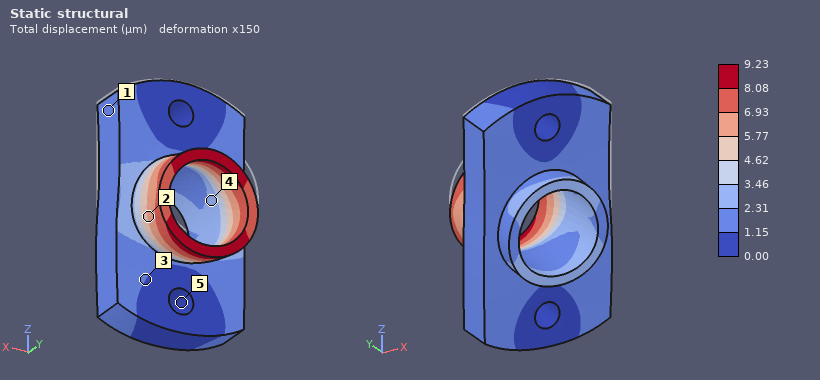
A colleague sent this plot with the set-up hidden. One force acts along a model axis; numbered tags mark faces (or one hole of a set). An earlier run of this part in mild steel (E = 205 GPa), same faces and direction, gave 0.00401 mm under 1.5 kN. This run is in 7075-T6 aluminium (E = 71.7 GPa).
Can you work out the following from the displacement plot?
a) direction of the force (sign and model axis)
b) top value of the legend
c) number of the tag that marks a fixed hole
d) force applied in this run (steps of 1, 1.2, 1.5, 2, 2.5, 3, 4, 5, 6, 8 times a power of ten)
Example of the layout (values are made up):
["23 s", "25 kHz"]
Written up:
["-Z", "9.23 µm", "5", "1.2 kN"]
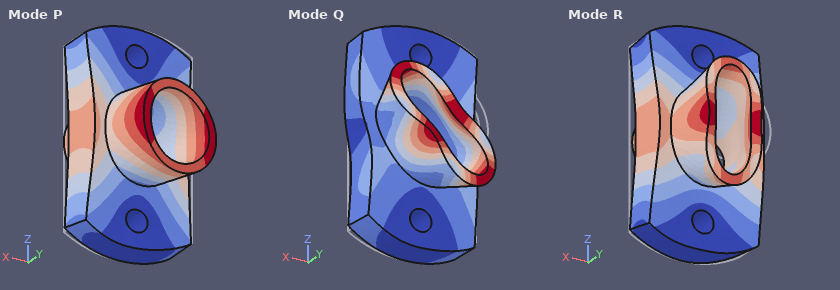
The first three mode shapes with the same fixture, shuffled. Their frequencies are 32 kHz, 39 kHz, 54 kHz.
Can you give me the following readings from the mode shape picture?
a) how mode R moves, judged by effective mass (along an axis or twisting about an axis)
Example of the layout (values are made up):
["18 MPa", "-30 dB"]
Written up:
["along Y"]
